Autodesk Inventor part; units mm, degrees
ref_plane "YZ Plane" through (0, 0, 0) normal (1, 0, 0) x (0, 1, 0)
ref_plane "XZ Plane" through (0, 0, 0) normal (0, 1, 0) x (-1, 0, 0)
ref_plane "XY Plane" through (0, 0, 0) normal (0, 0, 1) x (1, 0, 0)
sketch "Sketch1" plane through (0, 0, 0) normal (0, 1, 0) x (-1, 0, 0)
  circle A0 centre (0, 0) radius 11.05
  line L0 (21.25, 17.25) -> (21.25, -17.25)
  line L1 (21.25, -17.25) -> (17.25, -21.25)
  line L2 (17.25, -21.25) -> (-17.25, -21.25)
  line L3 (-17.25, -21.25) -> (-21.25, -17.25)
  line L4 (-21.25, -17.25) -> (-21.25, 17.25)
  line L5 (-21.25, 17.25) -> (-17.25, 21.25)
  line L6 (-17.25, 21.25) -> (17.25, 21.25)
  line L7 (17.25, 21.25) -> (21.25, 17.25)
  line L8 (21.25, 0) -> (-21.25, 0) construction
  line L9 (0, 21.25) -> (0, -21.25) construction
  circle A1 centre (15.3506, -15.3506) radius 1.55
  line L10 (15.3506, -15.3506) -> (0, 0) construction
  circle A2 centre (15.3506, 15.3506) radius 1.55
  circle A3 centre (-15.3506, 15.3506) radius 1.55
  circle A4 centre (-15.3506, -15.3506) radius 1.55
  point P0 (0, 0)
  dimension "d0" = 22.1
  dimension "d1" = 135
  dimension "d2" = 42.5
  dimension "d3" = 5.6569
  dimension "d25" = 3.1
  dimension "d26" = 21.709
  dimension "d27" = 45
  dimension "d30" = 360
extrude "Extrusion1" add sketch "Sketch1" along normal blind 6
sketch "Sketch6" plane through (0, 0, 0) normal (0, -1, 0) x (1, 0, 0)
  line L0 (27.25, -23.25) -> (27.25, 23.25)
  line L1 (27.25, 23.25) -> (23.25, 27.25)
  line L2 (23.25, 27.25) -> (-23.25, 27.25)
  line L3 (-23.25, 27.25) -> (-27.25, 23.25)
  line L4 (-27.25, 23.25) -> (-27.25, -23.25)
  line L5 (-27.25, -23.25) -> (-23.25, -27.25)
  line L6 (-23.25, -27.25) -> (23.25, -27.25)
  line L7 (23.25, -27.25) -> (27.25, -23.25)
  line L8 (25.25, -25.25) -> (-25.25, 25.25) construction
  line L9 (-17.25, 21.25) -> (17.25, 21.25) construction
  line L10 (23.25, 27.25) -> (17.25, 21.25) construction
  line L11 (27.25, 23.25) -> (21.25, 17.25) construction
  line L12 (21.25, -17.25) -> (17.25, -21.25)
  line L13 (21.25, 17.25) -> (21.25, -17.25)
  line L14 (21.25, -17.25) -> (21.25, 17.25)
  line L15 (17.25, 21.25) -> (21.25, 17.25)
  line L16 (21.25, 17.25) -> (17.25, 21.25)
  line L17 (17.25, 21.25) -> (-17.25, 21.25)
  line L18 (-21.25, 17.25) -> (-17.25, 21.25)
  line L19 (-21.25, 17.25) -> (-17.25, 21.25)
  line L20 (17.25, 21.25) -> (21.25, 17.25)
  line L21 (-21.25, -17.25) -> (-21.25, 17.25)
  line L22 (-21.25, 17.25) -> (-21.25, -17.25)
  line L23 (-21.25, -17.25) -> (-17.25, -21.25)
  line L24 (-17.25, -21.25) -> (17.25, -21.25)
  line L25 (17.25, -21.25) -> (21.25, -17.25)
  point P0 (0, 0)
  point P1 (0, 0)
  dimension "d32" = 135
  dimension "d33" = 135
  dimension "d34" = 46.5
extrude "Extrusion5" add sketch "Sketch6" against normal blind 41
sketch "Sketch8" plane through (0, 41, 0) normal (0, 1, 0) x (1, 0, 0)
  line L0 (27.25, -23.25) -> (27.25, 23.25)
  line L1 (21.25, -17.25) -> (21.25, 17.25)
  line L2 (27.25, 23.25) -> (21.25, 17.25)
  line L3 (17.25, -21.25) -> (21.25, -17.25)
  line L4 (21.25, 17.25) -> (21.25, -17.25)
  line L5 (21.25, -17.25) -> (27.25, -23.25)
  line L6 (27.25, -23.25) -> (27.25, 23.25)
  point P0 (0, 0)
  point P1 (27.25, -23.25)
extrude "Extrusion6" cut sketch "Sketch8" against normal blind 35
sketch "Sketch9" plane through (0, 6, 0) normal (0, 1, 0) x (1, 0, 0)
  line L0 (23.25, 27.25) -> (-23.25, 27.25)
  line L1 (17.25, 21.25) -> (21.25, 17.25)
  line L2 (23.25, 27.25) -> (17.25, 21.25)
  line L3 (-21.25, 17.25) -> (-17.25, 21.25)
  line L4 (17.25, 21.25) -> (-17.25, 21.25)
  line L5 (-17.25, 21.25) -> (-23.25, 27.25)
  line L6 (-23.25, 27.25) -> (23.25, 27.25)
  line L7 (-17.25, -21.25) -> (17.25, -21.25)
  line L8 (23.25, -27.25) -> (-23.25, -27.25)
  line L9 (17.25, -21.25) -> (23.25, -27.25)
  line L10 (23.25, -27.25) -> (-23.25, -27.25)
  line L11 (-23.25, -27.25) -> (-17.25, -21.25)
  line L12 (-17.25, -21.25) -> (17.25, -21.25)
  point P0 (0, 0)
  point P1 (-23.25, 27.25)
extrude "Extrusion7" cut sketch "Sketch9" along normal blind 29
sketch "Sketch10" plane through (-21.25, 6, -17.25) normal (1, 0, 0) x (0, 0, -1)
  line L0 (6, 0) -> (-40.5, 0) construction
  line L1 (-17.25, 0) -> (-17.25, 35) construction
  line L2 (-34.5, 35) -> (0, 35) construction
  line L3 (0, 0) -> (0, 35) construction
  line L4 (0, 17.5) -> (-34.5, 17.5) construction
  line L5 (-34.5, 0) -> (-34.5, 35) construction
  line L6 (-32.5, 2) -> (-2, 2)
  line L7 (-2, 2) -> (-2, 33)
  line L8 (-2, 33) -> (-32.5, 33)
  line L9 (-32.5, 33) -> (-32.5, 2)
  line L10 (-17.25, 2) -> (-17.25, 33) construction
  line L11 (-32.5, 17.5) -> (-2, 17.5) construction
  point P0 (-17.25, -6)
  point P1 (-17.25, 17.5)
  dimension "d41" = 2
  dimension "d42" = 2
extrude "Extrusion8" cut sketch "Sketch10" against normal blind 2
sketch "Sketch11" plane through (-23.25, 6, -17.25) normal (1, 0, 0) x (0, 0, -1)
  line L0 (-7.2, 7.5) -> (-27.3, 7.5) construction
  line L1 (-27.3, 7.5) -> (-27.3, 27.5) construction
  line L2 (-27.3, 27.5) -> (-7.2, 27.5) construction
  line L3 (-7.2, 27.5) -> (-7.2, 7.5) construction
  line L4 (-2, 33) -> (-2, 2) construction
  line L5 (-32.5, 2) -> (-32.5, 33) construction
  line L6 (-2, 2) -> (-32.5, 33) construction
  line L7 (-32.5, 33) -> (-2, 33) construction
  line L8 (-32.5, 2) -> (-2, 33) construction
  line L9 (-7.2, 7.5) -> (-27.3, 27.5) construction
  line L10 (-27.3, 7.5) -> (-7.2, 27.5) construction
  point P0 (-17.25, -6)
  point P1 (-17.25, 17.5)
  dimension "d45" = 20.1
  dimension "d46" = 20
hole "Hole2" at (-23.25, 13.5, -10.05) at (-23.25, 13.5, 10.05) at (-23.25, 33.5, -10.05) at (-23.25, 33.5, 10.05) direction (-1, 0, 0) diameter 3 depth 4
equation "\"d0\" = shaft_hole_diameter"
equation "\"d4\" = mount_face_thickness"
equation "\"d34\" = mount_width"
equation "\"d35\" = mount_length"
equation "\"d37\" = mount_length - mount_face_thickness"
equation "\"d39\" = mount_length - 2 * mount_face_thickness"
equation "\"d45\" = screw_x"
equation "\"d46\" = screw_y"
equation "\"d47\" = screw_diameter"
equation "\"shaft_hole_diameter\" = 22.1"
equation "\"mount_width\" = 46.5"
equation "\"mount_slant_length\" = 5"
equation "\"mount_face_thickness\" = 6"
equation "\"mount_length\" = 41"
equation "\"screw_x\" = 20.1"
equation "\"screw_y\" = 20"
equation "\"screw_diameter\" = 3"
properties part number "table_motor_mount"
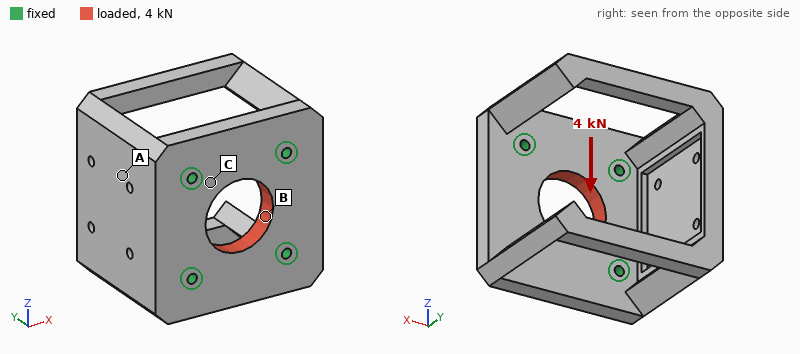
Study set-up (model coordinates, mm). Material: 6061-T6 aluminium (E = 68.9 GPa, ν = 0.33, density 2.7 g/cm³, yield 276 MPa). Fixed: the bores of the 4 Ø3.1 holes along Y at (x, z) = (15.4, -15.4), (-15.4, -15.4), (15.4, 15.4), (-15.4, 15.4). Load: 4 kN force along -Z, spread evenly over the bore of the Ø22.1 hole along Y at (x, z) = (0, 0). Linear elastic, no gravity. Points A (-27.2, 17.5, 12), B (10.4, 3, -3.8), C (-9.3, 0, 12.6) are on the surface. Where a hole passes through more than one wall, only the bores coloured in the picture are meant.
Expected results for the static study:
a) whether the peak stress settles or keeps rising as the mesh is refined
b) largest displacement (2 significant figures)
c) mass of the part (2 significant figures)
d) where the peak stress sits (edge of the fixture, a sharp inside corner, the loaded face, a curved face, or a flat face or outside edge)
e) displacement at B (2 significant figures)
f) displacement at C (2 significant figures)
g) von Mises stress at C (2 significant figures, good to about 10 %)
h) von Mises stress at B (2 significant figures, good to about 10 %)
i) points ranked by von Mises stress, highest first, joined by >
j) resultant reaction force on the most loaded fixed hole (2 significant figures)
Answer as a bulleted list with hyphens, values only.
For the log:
- keeps rising
- 4.2 µm
- 84 g
- edge of the fixture
- 2.5 µm
- 2.1 µm
- 10 MPa
- 17 MPa
- B > C > A
- 1.0 kN
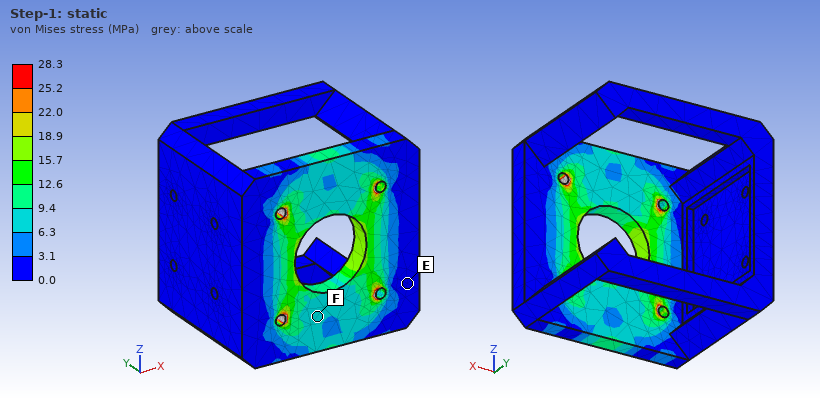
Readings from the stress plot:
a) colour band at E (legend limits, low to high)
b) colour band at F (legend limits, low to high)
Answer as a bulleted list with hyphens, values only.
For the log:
- 0.0 to 3.1 MPa
- 6.3 to 9.4 MPa
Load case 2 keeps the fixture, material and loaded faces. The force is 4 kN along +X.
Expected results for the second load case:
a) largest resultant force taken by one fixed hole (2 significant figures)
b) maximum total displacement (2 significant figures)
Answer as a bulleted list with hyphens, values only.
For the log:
- 1.0 kN
- 4.2 µm
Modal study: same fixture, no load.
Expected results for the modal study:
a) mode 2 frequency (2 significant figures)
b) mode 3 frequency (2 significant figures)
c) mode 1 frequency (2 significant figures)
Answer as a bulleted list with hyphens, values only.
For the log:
- 3000 Hz
- 3200 Hz
- 3000 Hz
